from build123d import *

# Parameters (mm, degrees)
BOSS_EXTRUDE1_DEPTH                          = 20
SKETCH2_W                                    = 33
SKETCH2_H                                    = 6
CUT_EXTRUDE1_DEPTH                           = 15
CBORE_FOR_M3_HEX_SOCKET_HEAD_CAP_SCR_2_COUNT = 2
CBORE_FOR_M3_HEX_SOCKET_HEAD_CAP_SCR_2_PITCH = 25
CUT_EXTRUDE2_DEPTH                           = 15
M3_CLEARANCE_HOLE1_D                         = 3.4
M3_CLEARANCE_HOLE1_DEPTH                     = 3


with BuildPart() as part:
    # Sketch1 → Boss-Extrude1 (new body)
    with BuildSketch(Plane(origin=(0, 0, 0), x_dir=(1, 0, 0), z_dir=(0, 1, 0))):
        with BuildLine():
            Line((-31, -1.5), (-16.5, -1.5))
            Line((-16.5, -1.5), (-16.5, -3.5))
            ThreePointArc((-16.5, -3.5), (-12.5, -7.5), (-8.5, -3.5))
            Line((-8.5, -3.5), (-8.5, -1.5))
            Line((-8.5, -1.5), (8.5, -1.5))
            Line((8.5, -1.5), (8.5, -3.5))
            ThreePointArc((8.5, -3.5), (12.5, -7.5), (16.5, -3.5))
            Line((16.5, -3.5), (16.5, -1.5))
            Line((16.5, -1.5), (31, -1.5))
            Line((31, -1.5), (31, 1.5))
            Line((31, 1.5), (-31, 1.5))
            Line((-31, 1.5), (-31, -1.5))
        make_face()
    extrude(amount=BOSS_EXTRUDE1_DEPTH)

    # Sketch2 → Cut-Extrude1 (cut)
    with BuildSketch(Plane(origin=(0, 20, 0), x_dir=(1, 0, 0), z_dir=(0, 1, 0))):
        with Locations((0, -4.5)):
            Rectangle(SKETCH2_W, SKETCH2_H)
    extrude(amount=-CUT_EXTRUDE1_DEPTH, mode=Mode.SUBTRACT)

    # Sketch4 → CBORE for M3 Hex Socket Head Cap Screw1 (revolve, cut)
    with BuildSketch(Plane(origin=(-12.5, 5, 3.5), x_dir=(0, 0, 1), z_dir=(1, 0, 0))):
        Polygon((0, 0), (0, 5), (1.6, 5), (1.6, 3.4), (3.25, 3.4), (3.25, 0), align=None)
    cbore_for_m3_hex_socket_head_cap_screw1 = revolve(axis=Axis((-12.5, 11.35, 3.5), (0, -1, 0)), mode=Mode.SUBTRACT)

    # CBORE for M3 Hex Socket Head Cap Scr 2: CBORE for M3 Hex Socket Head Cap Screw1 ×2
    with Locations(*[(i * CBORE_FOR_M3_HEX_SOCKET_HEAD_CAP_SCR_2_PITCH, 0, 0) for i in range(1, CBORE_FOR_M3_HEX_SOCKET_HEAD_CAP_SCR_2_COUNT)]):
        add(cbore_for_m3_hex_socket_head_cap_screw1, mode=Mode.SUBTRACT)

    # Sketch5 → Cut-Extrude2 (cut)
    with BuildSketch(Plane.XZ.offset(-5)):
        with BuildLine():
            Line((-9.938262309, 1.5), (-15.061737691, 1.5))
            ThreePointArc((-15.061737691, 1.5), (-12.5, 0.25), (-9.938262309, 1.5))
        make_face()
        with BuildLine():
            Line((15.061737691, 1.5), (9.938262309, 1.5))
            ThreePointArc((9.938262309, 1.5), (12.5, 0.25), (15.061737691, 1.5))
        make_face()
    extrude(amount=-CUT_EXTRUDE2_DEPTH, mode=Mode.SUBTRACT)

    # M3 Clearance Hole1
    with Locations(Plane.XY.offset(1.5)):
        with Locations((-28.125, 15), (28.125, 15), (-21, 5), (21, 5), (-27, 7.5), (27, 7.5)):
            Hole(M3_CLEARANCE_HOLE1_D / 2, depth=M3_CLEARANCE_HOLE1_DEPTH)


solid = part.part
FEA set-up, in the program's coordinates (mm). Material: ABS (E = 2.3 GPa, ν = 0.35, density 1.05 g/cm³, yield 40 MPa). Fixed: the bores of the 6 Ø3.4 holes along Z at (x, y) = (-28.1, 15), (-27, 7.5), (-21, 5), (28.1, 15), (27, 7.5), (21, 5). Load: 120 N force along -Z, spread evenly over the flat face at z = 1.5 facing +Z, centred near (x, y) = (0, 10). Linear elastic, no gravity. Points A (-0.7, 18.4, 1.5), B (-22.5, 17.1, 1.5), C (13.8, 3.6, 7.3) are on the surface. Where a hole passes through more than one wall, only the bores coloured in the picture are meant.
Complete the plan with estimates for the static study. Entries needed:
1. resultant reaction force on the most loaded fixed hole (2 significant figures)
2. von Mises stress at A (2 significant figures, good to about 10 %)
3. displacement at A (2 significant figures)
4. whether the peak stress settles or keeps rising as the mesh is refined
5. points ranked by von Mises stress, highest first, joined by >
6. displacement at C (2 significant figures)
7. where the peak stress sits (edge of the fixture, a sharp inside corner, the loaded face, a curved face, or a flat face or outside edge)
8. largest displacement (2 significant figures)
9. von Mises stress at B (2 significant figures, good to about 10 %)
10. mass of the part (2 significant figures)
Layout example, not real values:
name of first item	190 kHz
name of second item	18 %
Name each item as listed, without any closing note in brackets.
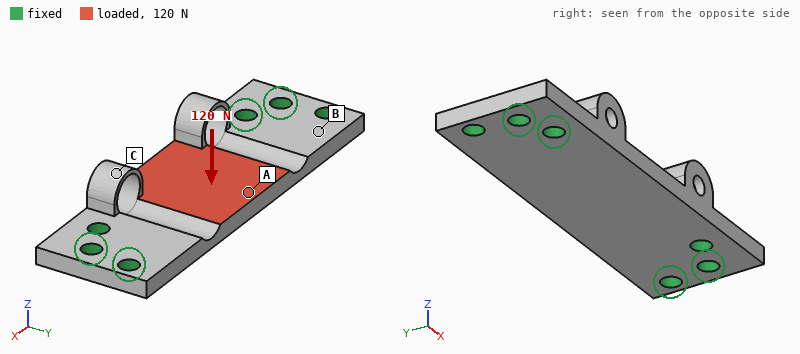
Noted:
resultant reaction force on the most loaded fixed hole	65 N
von Mises stress at A	14 MPa
displacement at A	0.62 mm
whether the peak stress settles or keeps rising as the mesh is refined	keeps rising
points ranked by von Mises stress, highest first, joined by >	A > B > C
displacement at C	0.21 mm
where the peak stress sits	edge of the fixture
largest displacement	0.66 mm
von Mises stress at B	10.0 MPa
mass of the part	3.8 g
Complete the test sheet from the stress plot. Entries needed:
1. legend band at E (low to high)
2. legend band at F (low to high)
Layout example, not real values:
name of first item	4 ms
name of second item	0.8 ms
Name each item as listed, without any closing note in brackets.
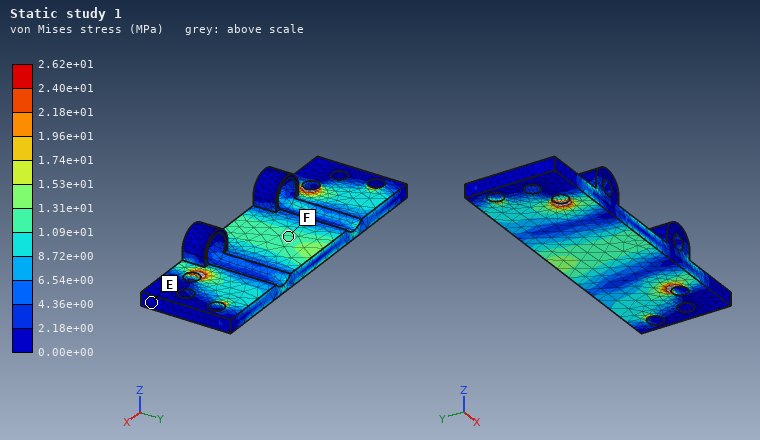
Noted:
legend band at E	0.00e+00 to 2.18e+00 MPa
legend band at F	1.09e+01 to 1.31e+01 MPa
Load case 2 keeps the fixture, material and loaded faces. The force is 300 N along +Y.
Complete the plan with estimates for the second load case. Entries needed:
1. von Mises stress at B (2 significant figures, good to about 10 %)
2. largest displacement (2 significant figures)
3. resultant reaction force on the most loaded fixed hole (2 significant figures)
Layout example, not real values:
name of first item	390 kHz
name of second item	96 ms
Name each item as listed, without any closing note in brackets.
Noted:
von Mises stress at B	3.5 MPa
largest displacement	0.40 mm
resultant reaction force on the most loaded fixed hole	180 N
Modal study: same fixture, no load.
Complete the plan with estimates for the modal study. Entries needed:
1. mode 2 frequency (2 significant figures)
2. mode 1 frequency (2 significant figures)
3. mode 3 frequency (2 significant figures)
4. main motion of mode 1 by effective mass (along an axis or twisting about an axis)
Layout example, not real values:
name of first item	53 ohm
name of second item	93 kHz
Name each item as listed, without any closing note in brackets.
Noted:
mode 2 frequency	3200 Hz
mode 1 frequency	2200 Hz
mode 3 frequency	5000 Hz
main motion of mode 1 by effective mass	along Z
